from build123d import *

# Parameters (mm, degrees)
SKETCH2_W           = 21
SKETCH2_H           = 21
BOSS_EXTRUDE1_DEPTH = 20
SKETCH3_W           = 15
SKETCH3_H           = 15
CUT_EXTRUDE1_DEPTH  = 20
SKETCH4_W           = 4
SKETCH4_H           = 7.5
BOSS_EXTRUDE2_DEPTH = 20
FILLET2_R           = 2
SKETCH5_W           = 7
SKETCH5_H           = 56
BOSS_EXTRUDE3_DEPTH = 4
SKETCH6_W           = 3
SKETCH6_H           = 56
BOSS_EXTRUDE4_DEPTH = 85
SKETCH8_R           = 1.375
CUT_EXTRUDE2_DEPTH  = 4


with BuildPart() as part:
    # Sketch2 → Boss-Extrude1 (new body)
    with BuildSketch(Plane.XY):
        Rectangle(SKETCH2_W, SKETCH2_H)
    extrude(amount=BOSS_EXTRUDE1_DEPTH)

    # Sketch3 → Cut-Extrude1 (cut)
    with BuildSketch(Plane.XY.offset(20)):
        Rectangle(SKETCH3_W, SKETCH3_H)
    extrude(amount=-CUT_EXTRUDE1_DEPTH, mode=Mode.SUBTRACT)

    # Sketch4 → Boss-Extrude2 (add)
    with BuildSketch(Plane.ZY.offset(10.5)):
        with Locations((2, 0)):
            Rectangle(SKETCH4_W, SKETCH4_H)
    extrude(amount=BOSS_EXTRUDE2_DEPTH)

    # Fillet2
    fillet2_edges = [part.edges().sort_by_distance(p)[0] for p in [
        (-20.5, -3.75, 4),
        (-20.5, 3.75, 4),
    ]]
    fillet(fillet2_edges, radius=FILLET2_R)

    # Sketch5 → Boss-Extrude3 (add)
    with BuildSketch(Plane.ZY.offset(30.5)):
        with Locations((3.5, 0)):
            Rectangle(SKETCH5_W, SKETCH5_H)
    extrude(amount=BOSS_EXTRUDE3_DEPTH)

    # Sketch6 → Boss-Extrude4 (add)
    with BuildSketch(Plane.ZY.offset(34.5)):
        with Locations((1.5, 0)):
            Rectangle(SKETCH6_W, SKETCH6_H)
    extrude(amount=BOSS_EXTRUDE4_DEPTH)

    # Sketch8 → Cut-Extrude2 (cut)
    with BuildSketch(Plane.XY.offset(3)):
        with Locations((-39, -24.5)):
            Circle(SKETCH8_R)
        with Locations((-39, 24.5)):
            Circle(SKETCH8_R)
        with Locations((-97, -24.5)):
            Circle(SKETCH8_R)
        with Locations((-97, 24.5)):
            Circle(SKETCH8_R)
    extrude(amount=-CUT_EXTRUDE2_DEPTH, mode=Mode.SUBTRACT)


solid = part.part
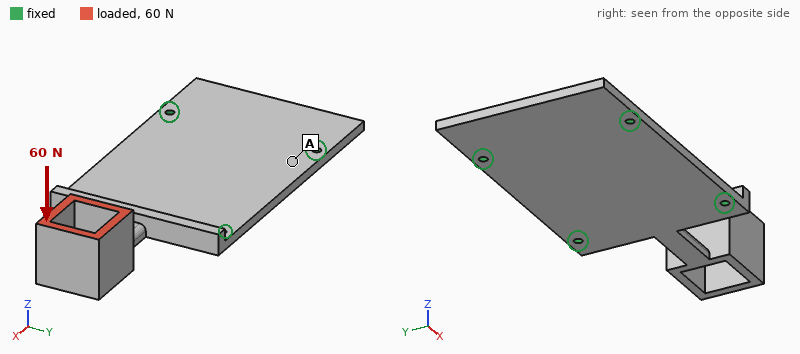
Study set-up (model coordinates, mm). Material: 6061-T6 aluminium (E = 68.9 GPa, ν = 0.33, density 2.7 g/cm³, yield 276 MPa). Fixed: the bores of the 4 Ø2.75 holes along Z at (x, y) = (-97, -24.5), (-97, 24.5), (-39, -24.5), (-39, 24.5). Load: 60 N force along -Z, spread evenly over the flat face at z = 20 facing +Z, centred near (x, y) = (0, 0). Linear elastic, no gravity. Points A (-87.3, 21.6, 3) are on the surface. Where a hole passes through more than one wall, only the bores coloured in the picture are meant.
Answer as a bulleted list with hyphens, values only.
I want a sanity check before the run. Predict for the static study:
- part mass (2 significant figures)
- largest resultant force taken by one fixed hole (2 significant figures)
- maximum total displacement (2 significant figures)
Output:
- 56 g
- 80 N
- 0.66 mm
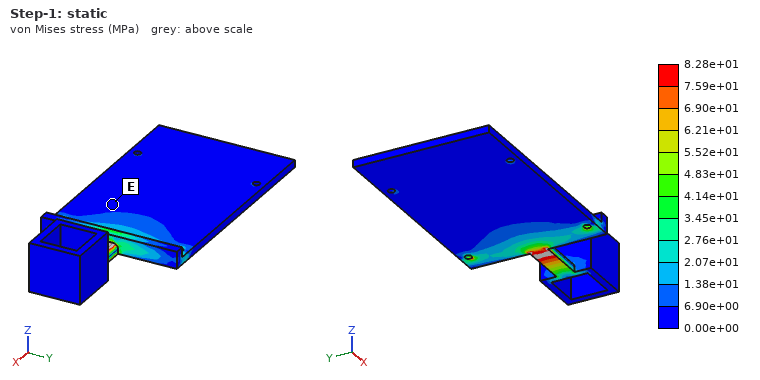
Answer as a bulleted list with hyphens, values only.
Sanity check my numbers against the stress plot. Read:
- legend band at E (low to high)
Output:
- 0.00e+00 to 6.90e+00 MPa
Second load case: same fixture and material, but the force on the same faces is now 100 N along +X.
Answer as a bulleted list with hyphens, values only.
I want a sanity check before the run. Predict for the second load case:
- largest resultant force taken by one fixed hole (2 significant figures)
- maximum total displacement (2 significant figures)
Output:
- 41 N
- 0.82 mm
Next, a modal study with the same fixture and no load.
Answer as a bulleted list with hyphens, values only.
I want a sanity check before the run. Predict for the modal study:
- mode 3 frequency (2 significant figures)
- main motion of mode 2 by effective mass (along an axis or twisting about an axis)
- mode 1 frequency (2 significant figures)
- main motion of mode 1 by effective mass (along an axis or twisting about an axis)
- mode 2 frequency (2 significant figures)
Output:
- 1800 Hz
- along Y
- 500 Hz
- along Z
- 920 Hz
